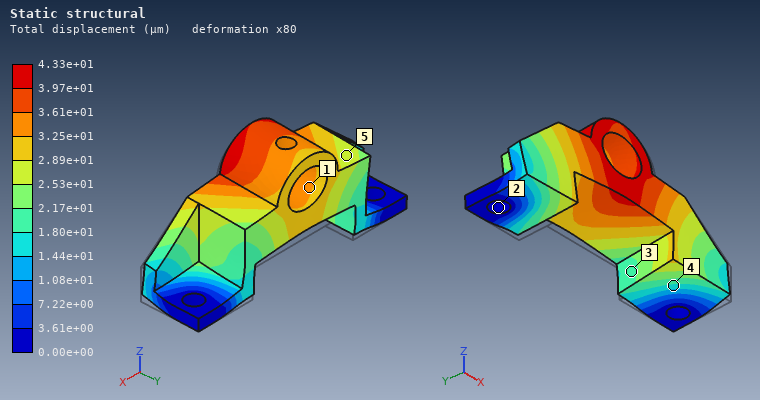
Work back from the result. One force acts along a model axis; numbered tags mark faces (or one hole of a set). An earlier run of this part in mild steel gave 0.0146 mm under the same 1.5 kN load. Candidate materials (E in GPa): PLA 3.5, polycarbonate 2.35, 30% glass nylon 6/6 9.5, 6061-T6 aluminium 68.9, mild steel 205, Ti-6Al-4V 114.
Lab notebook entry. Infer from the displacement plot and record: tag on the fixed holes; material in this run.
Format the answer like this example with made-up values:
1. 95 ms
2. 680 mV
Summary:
1. 2
2. 6061-T6 aluminium
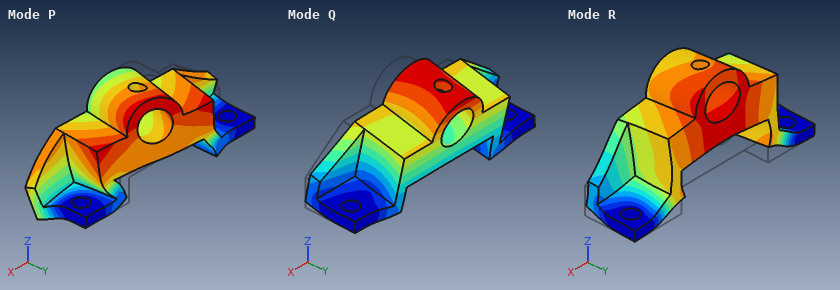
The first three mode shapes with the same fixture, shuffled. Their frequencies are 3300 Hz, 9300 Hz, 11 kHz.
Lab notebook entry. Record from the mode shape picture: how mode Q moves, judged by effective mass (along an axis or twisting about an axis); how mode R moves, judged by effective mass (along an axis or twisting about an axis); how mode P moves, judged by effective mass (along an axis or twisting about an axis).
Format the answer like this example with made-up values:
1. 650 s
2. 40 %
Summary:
1. along Y
2. along Z
3. along X
